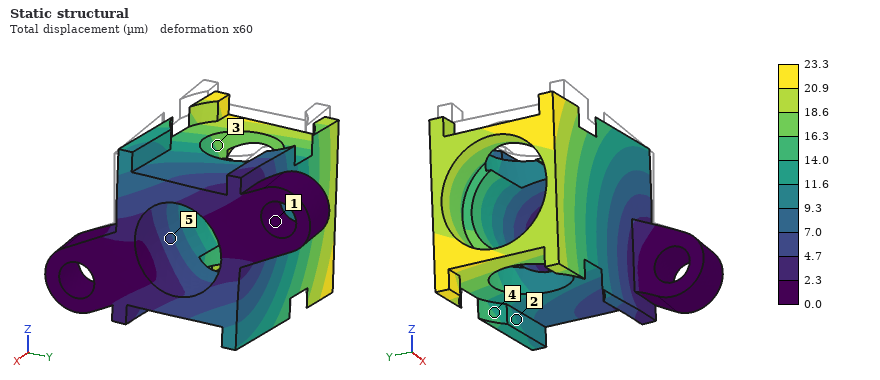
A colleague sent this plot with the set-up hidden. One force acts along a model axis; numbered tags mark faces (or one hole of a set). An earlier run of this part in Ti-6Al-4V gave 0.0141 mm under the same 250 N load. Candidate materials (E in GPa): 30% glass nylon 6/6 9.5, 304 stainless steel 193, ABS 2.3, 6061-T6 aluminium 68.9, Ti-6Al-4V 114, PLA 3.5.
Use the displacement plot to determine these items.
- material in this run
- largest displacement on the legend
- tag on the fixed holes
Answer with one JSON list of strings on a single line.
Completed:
["6061-T6 aluminium", "23.3 µm", "1"]
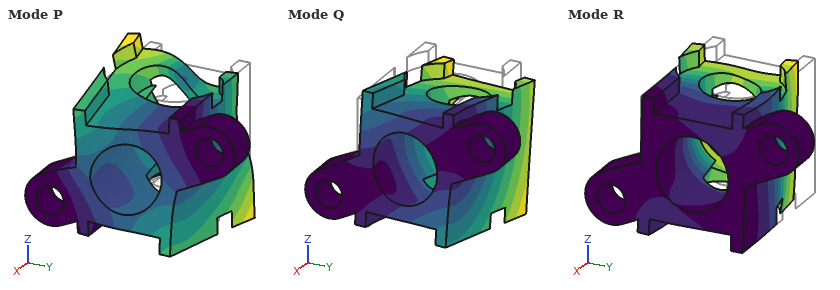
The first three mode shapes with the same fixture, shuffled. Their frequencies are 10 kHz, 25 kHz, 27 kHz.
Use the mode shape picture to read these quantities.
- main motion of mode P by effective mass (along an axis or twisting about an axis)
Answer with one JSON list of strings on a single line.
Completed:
["along X"]
